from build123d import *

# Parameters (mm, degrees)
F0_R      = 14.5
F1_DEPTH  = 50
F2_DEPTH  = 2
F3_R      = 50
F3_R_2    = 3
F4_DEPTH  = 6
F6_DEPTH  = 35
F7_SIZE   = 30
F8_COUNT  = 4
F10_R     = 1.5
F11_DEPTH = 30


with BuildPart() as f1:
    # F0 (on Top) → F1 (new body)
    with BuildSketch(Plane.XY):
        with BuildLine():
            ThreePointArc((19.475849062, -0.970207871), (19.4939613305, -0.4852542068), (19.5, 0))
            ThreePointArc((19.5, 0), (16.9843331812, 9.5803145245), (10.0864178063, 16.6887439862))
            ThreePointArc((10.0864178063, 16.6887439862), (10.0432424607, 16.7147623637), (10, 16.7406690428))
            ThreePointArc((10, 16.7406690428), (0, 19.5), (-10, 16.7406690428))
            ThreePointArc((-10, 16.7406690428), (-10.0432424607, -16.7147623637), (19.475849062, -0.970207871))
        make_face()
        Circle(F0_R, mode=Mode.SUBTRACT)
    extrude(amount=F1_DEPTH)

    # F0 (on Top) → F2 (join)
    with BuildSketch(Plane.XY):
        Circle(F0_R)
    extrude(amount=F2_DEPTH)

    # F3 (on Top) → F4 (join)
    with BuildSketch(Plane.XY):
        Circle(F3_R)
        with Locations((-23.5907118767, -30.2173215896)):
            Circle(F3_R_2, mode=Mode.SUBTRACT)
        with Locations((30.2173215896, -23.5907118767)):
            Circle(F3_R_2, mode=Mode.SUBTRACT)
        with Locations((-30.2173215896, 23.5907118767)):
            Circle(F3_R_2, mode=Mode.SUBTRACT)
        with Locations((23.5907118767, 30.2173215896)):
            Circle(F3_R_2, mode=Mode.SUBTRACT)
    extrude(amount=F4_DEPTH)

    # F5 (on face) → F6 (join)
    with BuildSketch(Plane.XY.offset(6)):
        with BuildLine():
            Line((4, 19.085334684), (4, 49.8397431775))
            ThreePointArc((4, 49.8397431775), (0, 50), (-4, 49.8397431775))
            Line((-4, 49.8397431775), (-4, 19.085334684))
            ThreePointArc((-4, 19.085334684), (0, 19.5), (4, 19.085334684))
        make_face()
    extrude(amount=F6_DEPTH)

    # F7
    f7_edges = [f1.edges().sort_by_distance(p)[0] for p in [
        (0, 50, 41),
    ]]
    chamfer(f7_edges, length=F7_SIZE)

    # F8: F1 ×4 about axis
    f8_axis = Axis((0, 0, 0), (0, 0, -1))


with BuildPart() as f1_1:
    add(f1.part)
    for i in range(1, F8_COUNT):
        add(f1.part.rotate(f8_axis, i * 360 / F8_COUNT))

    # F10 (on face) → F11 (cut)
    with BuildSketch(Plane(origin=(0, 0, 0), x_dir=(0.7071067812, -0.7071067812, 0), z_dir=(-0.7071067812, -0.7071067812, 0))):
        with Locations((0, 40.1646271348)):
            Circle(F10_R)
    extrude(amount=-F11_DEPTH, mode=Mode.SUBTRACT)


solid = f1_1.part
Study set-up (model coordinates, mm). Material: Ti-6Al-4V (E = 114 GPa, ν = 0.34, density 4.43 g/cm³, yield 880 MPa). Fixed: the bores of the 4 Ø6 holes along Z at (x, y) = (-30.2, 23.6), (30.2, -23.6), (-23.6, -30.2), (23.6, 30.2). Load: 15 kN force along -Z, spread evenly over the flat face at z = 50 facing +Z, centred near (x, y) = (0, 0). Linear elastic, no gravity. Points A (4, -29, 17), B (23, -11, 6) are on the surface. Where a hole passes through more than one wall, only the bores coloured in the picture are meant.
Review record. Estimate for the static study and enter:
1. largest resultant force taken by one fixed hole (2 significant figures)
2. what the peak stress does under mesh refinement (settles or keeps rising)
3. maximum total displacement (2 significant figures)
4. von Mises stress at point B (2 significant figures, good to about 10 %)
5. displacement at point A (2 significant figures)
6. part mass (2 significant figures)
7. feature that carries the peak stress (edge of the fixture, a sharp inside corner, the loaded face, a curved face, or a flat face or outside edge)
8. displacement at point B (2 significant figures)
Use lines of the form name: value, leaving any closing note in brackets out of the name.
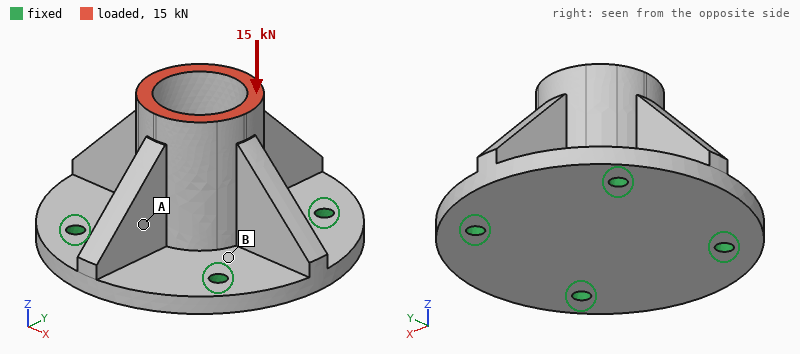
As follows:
largest resultant force taken by one fixed hole: 3.8 kN
what the peak stress does under mesh refinement: keeps rising
maximum total displacement: 48 µm
von Mises stress at point B: 48 MPa
displacement at point A: 39 µm
part mass: 400 g
feature that carries the peak stress: edge of the fixture
displacement at point B: 28 µm
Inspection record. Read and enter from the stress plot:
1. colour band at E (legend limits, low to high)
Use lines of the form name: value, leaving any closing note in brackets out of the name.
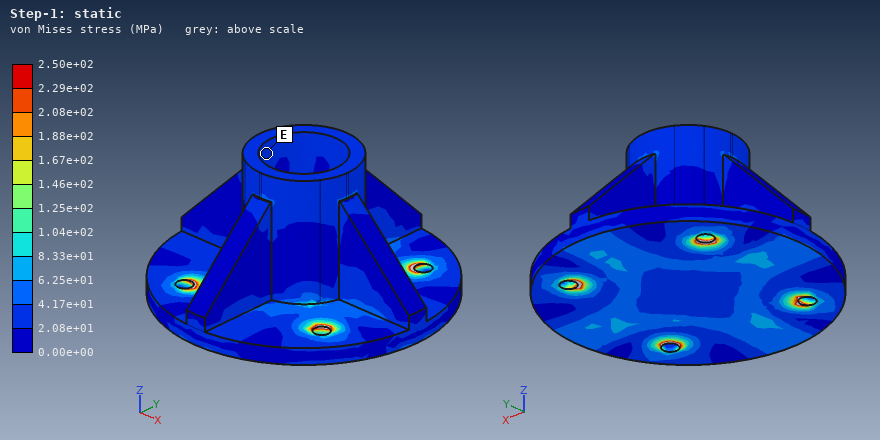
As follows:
colour band at E: 2.08e+01 to 4.17e+01 MPa
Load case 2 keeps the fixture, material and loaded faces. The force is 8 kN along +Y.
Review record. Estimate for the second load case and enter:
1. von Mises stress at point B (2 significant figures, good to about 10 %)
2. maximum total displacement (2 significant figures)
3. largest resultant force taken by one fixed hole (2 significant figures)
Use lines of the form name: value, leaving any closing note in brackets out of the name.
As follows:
von Mises stress at point B: 58 MPa
maximum total displacement: 0.12 mm
largest resultant force taken by one fixed hole: 4.5 kN
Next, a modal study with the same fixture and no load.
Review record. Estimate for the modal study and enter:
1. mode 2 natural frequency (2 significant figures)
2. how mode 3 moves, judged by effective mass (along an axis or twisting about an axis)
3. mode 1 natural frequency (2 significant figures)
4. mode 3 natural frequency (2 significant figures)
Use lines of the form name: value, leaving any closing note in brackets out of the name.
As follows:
mode 2 natural frequency: 4800 Hz
how mode 3 moves, judged by effective mass: along Z
mode 1 natural frequency: 4800 Hz
mode 3 natural frequency: 5600 Hz
